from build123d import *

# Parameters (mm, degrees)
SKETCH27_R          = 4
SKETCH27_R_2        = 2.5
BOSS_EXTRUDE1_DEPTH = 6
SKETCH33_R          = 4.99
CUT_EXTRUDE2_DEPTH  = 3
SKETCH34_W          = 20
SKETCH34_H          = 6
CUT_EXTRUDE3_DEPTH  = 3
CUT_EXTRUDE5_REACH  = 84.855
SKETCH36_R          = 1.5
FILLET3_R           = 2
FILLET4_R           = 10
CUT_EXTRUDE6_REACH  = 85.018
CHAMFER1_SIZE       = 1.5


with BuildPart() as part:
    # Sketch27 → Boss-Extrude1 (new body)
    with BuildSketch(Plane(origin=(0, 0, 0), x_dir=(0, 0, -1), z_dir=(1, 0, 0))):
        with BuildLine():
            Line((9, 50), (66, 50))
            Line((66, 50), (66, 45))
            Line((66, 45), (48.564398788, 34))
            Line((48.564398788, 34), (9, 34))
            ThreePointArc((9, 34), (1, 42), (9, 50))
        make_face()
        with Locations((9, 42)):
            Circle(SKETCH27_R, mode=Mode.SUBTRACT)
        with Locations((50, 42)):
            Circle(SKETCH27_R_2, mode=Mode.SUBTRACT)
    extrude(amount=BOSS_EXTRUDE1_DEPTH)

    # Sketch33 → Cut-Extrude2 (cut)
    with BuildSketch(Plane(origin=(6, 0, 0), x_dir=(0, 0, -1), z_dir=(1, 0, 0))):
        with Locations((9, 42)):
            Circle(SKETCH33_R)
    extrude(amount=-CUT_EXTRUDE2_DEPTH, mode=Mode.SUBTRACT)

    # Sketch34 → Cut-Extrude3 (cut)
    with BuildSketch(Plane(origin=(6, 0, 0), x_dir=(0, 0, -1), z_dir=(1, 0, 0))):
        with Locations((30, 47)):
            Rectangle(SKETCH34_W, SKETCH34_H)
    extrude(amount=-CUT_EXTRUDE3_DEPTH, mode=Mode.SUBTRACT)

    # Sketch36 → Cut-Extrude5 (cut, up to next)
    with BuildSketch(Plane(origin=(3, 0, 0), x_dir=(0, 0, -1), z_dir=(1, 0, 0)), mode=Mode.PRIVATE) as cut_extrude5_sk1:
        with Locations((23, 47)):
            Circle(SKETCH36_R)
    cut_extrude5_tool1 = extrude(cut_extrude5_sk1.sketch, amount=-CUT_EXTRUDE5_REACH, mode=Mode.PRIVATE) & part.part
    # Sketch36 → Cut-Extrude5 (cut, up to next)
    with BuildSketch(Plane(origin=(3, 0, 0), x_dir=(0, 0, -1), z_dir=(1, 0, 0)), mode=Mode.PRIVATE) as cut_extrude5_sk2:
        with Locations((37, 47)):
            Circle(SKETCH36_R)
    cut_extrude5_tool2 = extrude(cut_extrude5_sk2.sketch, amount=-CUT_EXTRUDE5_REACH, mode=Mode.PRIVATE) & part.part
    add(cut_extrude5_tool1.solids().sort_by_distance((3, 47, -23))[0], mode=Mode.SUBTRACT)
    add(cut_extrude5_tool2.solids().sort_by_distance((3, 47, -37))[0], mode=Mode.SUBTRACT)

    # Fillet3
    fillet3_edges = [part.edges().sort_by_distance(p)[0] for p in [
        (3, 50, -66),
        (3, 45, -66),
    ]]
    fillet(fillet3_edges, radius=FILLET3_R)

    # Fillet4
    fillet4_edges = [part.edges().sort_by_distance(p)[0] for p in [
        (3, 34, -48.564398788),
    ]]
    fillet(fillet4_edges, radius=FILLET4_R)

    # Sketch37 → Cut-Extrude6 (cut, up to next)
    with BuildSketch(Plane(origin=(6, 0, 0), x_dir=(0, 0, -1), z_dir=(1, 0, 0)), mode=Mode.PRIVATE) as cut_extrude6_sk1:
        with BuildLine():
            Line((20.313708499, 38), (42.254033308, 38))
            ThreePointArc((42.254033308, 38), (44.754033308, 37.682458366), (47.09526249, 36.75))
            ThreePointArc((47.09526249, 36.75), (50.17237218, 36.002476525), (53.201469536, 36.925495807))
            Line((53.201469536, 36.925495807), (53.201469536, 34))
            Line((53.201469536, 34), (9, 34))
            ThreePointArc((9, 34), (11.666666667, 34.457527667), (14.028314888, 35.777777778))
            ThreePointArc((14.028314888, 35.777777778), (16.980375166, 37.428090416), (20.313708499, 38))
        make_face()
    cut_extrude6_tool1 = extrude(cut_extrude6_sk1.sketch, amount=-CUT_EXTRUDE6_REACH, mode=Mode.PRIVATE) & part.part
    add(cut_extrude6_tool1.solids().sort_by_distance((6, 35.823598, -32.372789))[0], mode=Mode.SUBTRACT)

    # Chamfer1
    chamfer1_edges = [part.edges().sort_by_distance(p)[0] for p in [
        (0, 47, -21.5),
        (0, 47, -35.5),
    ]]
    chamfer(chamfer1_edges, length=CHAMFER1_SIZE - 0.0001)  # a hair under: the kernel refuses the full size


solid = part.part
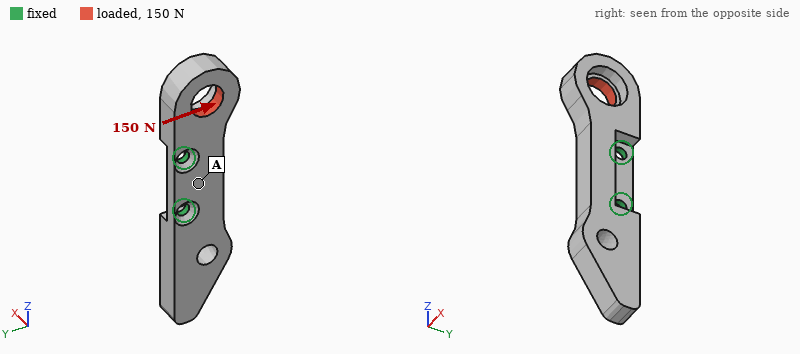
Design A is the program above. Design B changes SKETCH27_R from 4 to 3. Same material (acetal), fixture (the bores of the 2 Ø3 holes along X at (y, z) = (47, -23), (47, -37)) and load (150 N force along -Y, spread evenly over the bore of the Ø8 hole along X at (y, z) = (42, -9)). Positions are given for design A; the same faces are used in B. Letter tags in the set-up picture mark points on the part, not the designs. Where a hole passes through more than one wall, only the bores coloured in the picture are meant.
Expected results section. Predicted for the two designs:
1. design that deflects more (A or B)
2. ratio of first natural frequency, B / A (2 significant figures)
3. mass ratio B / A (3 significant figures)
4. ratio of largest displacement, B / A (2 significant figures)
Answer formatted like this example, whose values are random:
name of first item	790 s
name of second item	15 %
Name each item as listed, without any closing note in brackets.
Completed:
design that deflects more	A
ratio of first natural frequency, B / A	1.00
mass ratio B / A	1.02
ratio of largest displacement, B / A	0.92
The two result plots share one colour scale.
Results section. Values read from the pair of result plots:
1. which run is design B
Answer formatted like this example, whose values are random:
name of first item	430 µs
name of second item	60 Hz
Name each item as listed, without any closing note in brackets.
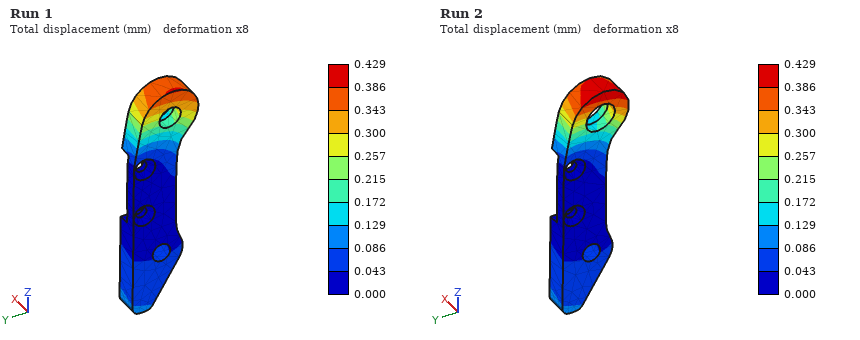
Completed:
which run is design B	Run 1
